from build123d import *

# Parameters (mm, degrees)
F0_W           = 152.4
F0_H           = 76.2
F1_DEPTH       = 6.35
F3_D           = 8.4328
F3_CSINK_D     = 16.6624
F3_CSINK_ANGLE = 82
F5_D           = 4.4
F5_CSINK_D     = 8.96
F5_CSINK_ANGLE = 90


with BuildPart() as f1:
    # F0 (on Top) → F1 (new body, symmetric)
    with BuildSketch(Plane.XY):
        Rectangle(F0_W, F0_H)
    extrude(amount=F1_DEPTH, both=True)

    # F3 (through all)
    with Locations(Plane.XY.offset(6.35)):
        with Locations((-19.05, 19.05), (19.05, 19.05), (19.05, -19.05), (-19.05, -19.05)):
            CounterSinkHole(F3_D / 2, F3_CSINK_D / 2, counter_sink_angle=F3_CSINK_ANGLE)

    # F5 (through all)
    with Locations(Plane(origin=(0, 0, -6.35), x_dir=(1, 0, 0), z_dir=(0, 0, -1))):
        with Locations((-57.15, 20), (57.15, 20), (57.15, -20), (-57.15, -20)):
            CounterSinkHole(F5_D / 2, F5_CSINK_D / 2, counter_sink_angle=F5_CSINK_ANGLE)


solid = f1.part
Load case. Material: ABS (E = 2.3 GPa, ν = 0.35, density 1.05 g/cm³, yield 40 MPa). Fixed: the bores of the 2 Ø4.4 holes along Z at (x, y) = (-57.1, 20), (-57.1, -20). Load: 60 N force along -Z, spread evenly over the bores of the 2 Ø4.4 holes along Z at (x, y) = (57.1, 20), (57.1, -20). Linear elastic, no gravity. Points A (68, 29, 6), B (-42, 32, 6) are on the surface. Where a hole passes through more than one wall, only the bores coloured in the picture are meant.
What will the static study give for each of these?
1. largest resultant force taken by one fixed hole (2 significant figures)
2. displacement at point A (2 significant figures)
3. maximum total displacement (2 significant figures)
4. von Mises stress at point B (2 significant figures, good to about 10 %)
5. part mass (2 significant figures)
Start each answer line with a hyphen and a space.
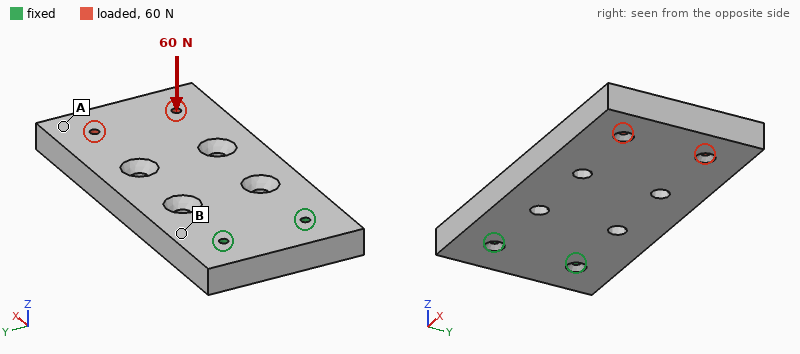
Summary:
- 31 N
- 1.5 mm
- 1.7 mm
- 2.8 MPa
- 150 g
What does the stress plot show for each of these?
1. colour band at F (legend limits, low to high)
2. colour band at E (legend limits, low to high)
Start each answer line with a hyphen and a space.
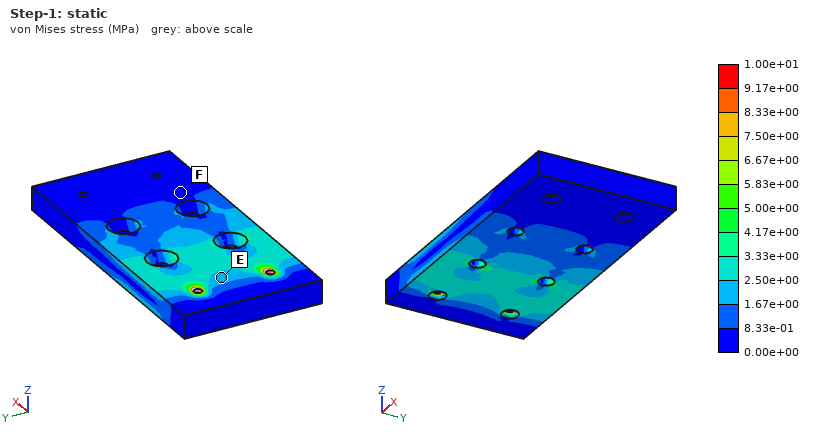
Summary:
- 0.00e+00 to 8.33e-01 MPa
- 1.67e+00 to 2.50e+00 MPa
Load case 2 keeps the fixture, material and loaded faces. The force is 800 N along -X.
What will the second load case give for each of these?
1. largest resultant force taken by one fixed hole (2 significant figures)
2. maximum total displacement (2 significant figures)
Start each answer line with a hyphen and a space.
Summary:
- 400 N
- 0.33 mm
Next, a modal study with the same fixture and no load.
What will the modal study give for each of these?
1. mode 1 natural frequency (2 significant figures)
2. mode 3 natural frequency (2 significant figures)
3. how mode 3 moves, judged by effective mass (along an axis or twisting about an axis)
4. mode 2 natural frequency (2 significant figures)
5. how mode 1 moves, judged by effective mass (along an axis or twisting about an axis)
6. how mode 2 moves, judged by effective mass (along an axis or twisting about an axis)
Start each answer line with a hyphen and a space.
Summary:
- 150 Hz
- 660 Hz
- along Y
- 550 Hz
- along Z
- twisting about X
